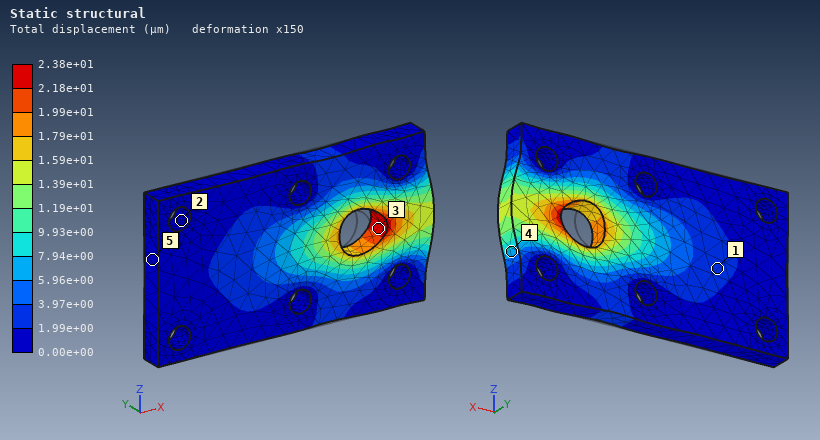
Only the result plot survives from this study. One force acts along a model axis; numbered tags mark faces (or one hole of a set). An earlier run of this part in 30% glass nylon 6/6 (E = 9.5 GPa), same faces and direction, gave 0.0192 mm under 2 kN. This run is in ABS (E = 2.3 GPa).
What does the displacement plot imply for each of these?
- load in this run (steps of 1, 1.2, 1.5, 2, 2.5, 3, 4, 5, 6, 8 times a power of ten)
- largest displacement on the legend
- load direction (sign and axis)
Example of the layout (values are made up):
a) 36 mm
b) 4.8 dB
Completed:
a) 600 N
b) 2.38e+01 µm
c) +X
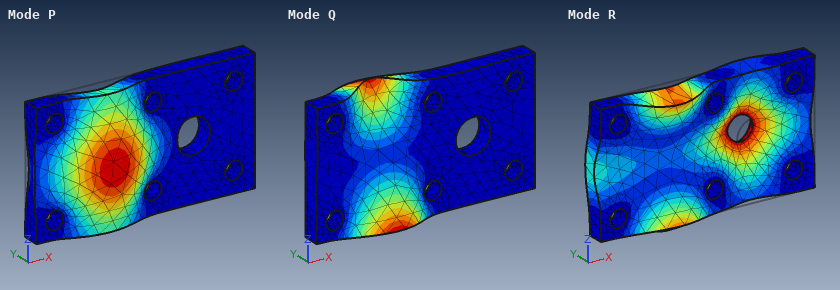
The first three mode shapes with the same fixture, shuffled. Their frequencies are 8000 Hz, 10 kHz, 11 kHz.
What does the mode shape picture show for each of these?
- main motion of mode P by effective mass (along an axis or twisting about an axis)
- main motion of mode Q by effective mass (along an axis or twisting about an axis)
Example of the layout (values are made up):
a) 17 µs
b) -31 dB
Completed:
a) along Y
b) twisting about X
